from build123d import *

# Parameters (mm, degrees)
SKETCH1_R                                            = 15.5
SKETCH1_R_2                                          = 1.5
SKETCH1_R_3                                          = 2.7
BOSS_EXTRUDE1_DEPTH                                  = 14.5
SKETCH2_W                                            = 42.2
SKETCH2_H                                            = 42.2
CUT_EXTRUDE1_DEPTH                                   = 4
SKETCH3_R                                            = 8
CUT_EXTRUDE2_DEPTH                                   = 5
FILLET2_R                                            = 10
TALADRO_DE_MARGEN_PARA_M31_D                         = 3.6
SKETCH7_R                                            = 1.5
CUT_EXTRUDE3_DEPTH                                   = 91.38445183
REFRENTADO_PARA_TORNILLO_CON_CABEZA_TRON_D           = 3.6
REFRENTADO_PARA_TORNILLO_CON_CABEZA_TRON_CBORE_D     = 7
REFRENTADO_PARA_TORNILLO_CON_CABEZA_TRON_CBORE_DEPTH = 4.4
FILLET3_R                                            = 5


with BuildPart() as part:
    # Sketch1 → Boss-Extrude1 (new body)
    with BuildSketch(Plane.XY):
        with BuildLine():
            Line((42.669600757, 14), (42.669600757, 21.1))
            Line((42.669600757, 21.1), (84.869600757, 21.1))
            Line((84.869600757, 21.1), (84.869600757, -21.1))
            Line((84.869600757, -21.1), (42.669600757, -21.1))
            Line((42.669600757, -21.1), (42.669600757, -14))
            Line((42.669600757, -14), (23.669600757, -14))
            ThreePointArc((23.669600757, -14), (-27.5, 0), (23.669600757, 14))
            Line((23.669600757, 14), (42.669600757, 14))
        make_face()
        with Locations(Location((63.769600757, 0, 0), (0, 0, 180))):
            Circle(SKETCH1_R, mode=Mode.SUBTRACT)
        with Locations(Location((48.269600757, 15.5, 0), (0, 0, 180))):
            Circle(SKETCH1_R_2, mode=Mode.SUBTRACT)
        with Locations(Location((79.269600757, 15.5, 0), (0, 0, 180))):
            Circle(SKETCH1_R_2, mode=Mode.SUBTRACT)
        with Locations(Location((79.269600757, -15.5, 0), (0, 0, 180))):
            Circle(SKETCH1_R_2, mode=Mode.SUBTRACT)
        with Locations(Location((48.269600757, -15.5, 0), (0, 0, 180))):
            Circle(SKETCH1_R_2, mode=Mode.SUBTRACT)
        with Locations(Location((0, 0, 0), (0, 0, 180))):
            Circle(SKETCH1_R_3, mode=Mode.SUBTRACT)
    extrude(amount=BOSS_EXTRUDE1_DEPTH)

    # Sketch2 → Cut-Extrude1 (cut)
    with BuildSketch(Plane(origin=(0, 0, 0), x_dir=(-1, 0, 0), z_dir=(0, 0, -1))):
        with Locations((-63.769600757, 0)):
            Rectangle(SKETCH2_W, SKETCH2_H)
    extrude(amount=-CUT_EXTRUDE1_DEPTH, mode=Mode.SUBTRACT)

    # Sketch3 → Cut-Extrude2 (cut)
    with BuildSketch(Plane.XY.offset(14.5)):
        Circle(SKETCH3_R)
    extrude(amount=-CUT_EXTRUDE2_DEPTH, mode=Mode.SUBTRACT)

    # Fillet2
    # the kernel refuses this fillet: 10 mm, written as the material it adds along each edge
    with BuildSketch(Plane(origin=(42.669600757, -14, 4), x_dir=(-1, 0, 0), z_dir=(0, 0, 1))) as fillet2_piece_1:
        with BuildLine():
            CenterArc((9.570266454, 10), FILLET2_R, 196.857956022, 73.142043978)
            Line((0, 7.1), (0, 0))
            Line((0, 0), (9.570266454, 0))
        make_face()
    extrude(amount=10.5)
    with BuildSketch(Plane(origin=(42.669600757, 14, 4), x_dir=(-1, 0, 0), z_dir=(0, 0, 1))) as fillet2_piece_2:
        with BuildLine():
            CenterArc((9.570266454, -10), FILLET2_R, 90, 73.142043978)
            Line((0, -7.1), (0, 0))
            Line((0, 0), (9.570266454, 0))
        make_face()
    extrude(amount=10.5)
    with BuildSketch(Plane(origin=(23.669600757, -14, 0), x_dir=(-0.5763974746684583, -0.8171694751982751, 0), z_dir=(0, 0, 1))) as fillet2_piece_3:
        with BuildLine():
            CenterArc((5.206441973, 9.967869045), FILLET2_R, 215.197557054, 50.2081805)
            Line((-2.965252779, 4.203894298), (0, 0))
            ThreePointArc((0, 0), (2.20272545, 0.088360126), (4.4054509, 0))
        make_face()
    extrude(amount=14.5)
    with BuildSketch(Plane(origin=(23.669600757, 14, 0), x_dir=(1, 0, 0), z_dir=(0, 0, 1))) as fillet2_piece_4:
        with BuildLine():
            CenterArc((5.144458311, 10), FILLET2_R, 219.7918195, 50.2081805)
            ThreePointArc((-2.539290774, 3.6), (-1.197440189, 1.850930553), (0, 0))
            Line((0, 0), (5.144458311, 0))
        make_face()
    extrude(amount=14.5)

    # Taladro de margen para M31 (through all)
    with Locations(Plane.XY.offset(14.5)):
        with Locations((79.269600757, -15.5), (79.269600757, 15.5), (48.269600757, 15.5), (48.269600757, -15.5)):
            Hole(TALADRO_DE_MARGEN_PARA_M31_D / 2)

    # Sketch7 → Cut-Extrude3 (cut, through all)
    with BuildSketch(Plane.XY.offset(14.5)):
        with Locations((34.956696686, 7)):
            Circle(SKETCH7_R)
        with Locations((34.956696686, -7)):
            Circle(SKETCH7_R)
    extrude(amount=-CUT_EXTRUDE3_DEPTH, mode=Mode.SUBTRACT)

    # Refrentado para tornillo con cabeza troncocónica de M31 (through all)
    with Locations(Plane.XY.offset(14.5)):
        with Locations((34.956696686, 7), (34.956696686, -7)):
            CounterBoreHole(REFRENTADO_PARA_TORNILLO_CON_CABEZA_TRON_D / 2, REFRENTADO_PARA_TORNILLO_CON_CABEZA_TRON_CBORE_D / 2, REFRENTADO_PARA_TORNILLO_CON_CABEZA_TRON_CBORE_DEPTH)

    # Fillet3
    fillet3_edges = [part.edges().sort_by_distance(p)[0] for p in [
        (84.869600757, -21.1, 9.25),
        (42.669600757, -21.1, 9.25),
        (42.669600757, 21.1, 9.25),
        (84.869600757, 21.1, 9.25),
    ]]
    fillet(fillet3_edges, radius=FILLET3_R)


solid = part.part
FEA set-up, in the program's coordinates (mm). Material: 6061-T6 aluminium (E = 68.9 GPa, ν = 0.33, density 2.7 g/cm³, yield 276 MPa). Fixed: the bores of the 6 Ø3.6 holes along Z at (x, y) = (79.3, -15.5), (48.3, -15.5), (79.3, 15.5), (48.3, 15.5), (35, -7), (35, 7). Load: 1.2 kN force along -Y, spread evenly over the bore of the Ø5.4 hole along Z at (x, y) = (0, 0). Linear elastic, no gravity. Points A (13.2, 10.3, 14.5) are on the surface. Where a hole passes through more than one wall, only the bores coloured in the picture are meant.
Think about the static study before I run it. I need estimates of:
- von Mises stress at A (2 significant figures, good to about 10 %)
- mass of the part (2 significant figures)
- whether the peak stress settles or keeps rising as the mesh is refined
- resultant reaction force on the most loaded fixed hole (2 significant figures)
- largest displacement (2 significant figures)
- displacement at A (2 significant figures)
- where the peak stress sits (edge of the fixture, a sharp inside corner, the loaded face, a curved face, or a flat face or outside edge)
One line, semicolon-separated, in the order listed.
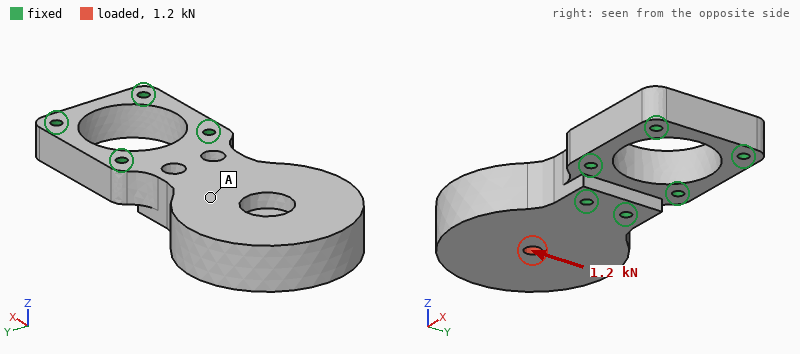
3.8 MPa; 140 g; keeps rising; 1.8 kN; 29 µm; 9.3 µm; edge of the fixture
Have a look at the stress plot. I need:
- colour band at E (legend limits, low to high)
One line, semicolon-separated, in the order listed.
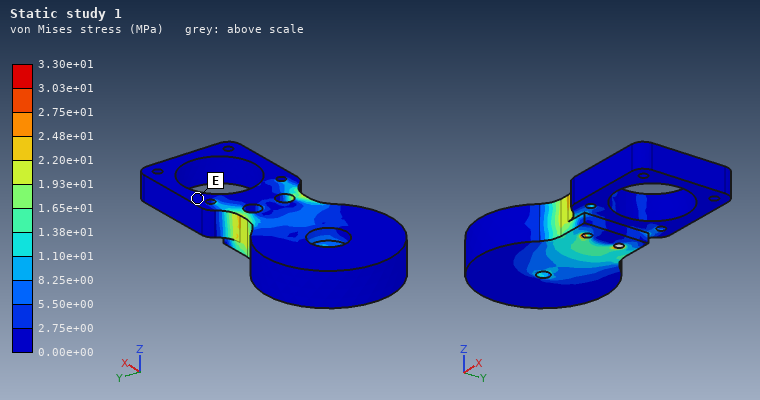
0.00e+00 to 2.75e+00 MPa
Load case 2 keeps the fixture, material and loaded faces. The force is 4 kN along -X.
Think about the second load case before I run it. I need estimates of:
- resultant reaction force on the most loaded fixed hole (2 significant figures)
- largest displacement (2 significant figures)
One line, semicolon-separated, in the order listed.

1.8 kN; 25 µm
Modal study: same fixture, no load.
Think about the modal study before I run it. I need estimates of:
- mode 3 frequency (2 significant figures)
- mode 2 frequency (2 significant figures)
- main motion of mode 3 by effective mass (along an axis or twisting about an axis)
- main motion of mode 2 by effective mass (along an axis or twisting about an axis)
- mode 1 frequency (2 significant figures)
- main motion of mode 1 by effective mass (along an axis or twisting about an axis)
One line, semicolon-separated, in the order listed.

5400 Hz; 4000 Hz; twisting about X; along Y; 2300 Hz; along Z
